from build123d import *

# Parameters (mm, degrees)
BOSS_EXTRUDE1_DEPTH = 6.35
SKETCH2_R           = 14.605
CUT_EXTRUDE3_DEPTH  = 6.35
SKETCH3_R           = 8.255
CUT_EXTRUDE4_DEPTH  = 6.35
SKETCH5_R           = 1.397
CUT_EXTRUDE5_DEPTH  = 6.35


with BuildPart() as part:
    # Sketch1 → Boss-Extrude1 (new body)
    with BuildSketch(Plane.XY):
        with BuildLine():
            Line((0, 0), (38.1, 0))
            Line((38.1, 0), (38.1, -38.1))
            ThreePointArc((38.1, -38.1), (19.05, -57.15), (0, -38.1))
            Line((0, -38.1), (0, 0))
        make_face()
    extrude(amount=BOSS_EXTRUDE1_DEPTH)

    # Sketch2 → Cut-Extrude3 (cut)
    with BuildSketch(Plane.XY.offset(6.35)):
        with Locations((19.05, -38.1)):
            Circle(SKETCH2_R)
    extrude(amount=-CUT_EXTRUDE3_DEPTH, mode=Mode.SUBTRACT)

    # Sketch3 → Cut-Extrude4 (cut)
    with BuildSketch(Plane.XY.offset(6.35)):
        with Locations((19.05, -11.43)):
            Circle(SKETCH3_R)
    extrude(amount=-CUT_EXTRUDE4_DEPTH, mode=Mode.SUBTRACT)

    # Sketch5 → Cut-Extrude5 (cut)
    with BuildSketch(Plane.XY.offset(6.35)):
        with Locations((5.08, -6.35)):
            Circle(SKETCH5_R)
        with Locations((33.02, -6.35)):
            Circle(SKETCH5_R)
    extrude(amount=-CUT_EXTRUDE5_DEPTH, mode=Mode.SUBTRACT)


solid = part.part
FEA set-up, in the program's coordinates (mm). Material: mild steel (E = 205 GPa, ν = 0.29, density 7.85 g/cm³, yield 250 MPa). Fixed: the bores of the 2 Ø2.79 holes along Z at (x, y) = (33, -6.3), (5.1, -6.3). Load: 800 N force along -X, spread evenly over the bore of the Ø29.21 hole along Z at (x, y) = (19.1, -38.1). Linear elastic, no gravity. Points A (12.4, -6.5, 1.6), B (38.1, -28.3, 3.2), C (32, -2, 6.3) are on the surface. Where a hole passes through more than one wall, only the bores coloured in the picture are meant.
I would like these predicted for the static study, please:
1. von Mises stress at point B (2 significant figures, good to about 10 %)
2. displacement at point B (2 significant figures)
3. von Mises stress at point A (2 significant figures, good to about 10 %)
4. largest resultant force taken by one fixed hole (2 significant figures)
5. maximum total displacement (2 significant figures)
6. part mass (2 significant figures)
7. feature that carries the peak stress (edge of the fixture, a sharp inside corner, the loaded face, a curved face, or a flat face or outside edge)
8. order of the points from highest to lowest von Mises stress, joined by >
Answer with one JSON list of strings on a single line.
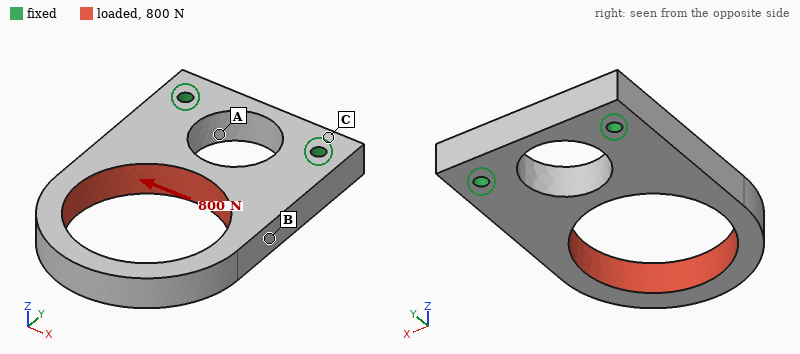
["48 MPa", "9.9 µm", "24 MPa", "810 N", "35 µm", "56 g", "edge of the fixture", "B > A > C"]
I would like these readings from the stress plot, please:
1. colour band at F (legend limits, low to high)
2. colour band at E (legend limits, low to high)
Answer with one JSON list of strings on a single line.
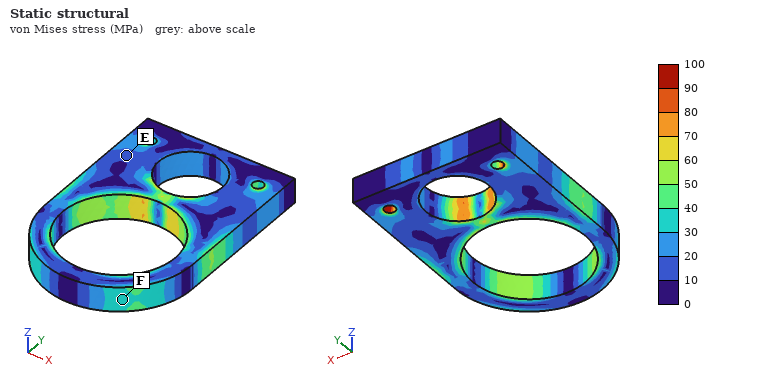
["30 to 40 MPa", "10 to 20 MPa"]
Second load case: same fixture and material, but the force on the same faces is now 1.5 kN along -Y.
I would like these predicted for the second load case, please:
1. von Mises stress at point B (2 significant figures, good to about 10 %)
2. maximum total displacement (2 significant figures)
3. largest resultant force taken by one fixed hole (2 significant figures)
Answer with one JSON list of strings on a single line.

["26 MPa", "8.5 µm", "750 N"]
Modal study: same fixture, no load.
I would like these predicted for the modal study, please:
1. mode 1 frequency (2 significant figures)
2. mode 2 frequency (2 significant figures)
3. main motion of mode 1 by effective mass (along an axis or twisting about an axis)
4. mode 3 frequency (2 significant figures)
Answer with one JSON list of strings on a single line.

["2400 Hz", "5500 Hz", "along Z", "5500 Hz"]
